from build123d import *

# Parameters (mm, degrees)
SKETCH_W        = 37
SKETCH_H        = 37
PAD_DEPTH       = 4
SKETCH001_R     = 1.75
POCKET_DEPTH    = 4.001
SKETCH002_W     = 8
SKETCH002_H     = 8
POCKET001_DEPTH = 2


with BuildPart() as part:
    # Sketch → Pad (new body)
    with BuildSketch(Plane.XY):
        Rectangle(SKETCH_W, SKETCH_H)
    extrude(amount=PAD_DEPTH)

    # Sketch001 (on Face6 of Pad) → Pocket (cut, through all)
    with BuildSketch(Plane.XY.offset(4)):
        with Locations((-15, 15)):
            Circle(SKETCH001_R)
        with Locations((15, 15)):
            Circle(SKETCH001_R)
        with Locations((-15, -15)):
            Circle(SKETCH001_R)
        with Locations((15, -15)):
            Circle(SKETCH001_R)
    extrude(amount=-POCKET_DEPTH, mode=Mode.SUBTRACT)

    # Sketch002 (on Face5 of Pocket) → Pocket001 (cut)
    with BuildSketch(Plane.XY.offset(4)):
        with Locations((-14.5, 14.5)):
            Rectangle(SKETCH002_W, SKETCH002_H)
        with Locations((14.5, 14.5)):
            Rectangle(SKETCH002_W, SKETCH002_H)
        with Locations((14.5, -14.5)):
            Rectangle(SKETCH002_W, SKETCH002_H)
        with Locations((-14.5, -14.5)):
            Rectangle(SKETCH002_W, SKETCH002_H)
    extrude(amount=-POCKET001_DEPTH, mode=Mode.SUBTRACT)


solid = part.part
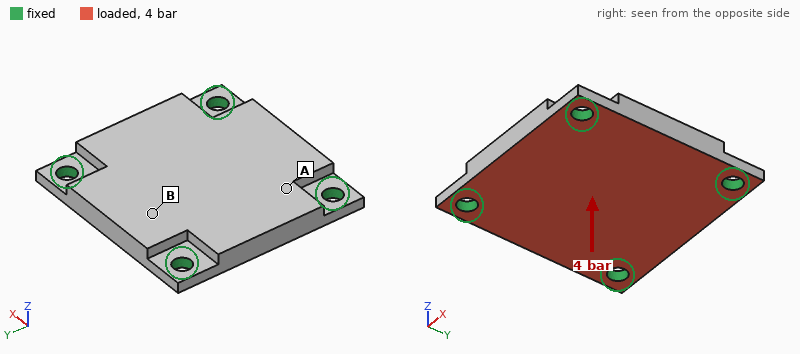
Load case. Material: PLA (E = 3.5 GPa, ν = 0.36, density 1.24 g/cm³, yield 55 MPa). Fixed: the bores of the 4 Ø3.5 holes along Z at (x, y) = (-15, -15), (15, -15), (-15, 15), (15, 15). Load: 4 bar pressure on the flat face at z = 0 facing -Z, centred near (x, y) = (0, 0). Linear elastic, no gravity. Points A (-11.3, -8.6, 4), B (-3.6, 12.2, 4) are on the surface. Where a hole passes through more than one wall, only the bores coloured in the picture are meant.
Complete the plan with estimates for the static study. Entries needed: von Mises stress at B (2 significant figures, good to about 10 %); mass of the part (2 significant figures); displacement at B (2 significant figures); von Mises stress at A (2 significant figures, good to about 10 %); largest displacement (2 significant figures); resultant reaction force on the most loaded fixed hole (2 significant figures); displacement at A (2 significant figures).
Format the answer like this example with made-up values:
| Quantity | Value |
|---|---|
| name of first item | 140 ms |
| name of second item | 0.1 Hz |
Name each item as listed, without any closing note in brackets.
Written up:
| Quantity | Value |
|---|---|
| von Mises stress at B | 8.7 MPa |
| mass of the part | 6.1 g |
| displacement at B | 0.12 mm |
| von Mises stress at A | 5.2 MPa |
| largest displacement | 0.17 mm |
| resultant reaction force on the most loaded fixed hole | 170 N |
| displacement at A | 0.093 mm |
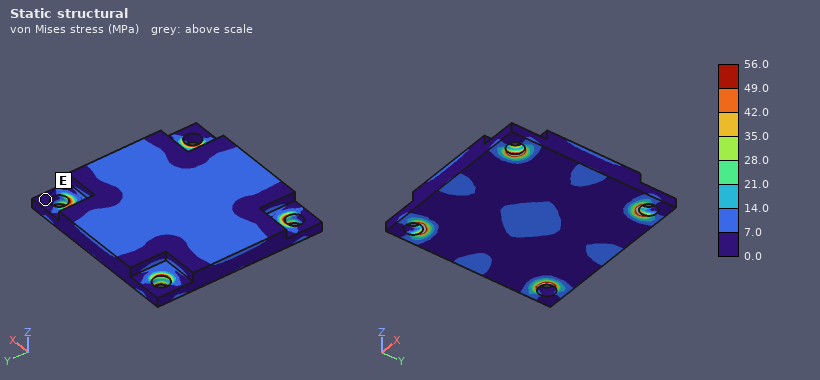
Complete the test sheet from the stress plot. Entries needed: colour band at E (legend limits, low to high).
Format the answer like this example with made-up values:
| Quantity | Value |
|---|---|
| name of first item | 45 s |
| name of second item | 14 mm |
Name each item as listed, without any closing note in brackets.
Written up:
| Quantity | Value |
|---|---|
| colour band at E | 0.0 to 7.0 MPa |
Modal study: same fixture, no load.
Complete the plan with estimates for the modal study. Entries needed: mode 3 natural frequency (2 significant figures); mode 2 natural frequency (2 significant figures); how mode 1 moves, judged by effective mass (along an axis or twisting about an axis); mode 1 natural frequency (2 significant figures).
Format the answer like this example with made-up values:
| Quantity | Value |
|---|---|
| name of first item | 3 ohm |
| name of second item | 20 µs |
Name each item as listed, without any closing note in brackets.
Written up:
| Quantity | Value |
|---|---|
| mode 3 natural frequency | 6300 Hz |
| mode 2 natural frequency | 6300 Hz |
| how mode 1 moves, judged by effective mass | along Z |
| mode 1 natural frequency | 4100 Hz |
